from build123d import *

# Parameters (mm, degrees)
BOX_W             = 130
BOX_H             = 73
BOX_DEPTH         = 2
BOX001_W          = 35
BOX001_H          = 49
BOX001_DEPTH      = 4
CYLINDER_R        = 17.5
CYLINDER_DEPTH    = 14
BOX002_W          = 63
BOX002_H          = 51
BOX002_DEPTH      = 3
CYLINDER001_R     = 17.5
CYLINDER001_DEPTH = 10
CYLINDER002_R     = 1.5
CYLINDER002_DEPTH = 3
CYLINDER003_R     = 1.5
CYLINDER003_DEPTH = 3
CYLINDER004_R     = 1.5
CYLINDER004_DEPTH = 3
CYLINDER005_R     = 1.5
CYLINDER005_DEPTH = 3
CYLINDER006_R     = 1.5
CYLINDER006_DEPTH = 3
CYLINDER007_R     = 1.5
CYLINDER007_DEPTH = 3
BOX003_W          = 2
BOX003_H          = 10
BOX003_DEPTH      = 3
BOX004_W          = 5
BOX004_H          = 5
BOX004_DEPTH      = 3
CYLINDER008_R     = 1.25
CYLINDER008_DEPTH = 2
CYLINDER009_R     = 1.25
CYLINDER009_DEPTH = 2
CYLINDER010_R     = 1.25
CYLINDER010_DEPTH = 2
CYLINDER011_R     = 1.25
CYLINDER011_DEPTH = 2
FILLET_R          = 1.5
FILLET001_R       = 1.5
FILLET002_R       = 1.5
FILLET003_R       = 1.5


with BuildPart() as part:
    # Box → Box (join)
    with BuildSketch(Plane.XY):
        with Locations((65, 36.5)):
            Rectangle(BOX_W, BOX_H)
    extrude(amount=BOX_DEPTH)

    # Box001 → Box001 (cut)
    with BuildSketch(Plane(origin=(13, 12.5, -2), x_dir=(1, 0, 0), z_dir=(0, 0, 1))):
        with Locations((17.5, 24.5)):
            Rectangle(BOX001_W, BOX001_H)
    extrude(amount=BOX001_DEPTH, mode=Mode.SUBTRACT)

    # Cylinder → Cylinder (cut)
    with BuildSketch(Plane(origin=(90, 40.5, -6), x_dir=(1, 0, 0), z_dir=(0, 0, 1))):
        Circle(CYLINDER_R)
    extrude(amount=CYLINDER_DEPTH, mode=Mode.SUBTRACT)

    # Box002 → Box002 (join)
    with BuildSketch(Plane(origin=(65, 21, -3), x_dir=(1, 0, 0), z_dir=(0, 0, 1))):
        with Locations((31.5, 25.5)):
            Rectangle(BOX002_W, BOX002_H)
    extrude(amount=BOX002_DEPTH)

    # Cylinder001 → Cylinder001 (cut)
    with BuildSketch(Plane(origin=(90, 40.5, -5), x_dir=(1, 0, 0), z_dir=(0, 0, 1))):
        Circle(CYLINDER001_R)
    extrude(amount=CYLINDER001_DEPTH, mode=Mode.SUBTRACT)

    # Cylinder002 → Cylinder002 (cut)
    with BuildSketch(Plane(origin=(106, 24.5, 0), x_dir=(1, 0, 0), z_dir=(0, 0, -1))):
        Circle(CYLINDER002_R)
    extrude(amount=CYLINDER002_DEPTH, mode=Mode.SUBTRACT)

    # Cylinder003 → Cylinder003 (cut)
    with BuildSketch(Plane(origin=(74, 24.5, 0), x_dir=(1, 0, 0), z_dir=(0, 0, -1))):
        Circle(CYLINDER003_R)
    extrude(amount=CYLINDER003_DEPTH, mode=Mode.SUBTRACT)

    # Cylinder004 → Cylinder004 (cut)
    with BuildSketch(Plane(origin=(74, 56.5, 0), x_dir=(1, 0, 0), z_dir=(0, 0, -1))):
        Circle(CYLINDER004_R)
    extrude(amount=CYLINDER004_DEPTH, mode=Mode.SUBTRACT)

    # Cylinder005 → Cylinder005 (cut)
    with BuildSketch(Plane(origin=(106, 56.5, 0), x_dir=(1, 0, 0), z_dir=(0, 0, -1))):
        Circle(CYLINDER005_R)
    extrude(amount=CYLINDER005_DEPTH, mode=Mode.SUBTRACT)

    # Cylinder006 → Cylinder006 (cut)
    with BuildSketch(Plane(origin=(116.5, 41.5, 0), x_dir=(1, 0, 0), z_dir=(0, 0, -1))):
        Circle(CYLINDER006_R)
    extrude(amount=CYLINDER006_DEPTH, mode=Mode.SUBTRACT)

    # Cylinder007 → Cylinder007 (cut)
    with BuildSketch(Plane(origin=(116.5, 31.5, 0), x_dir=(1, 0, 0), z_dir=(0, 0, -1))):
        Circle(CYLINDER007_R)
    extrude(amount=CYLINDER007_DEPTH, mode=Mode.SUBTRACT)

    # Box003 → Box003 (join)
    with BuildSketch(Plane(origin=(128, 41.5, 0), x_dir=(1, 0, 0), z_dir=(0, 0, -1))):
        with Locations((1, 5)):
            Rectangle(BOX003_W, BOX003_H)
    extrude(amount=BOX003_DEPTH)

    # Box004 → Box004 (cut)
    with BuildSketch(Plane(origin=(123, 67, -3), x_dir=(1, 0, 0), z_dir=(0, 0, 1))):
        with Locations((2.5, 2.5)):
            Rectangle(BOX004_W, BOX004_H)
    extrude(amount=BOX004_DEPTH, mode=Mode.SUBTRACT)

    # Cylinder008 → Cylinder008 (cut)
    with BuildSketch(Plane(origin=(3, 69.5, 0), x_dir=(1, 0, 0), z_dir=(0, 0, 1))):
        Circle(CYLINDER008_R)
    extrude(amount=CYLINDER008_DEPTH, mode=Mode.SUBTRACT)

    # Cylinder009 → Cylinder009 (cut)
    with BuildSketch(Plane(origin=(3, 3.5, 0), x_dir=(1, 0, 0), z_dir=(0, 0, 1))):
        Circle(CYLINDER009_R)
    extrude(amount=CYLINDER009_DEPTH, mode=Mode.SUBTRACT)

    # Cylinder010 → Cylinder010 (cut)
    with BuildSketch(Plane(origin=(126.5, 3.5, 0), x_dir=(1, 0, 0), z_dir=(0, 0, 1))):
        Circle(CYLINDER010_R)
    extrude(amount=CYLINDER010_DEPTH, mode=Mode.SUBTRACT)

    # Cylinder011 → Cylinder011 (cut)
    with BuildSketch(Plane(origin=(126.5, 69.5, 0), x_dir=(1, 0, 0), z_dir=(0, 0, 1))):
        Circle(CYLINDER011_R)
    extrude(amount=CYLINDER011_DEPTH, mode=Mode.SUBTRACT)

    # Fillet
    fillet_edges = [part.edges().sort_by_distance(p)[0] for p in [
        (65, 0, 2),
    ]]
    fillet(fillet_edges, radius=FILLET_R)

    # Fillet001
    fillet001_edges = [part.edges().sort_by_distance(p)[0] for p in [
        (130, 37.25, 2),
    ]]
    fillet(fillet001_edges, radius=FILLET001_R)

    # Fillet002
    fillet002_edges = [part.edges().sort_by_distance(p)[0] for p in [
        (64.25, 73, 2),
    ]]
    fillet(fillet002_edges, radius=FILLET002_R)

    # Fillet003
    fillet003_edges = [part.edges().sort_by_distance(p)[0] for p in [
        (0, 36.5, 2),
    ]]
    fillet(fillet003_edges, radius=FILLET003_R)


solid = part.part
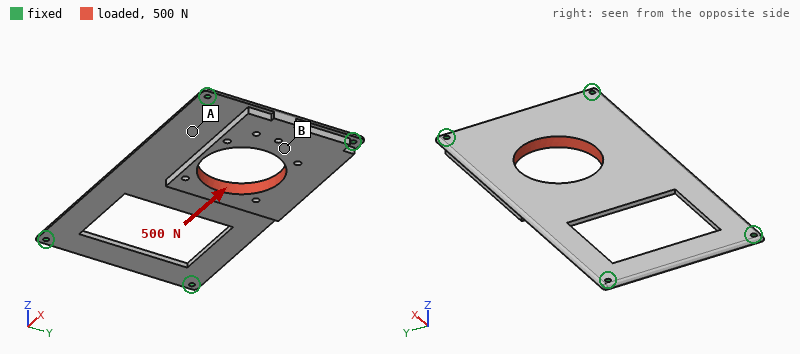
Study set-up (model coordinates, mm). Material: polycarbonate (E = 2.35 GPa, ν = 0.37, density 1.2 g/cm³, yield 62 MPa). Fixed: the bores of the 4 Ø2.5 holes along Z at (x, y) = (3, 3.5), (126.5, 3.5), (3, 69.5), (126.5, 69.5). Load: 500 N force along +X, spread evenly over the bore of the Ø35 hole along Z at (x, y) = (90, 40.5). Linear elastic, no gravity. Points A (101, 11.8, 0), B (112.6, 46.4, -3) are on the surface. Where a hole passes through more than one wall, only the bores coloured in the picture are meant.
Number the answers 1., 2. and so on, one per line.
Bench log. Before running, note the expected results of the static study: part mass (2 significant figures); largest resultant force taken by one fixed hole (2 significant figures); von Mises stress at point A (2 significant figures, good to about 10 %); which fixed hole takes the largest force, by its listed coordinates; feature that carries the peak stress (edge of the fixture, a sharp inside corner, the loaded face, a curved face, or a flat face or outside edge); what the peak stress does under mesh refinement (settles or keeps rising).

1. 24 g
2. 230 N
3. 3.1 MPa
4. (126.5, 69.5)
5. edge of the fixture
6. keeps rising
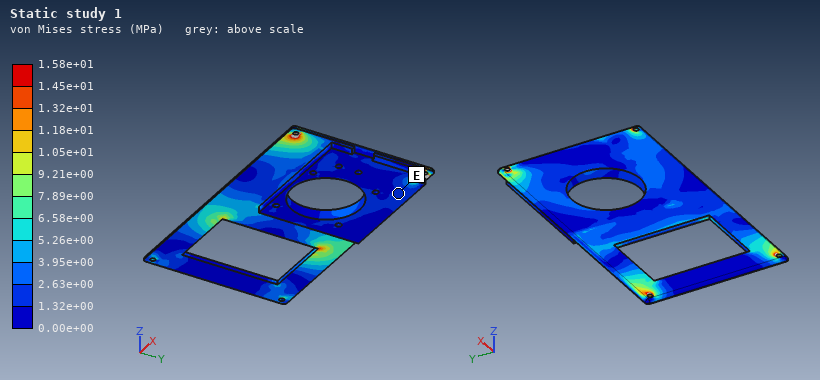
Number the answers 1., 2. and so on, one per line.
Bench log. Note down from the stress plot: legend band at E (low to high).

1. 1.32e+00 to 2.63e+00 MPa
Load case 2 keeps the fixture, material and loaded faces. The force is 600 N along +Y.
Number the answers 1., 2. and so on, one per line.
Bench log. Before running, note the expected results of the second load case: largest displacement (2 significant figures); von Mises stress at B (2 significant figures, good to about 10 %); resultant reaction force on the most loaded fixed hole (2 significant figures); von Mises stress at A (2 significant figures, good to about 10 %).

1. 0.49 mm
2. 4.5 MPa
3. 380 N
4. 8.1 MPa
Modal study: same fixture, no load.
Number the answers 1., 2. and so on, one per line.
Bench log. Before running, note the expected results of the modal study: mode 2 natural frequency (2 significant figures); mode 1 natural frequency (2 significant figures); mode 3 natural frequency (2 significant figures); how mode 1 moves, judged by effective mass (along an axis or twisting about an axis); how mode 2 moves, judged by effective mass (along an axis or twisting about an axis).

1. 340 Hz
2. 150 Hz
3. 590 Hz
4. along Z
5. twisting about X
